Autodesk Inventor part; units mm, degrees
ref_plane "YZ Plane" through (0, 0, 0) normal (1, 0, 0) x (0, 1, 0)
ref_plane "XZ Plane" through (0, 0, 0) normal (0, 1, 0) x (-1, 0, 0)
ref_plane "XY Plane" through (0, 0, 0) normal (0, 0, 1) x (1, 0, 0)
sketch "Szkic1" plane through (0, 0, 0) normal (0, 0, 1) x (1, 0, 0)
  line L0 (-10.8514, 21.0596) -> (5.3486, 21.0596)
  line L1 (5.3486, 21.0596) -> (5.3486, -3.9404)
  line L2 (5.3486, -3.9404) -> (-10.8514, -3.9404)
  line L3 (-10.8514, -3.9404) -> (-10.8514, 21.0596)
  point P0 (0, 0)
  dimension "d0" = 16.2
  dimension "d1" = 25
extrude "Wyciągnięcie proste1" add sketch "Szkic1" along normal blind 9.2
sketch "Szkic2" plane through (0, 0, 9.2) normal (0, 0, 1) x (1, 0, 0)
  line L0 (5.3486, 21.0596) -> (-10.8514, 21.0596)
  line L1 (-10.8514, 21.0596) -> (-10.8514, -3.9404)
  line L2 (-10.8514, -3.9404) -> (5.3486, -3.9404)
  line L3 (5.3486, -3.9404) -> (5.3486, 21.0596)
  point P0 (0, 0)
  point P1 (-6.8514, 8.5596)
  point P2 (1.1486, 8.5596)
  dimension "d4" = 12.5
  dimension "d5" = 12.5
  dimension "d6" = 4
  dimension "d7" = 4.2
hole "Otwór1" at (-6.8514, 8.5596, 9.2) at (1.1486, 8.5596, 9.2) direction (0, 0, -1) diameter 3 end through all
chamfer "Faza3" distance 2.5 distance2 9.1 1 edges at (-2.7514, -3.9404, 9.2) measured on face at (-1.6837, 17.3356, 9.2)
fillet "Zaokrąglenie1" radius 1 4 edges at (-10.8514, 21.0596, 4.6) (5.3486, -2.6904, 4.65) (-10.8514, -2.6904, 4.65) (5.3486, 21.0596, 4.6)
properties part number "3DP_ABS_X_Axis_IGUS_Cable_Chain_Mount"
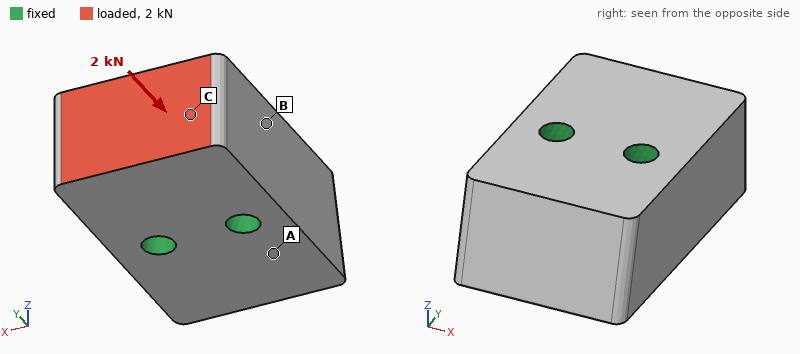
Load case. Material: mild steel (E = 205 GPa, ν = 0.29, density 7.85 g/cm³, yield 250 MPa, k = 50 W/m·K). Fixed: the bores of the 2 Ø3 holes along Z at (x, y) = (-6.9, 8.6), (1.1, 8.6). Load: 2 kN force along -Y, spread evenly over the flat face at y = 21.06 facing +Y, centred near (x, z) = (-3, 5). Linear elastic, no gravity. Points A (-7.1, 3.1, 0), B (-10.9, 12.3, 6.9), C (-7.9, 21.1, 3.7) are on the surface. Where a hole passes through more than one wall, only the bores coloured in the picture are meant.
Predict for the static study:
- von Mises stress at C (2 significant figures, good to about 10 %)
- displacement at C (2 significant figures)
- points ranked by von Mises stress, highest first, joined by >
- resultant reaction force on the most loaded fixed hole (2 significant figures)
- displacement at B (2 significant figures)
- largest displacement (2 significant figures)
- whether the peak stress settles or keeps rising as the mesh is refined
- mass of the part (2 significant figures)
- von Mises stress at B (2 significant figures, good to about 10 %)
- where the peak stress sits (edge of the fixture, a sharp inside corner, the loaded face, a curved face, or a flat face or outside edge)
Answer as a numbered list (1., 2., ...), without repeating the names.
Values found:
1. 12 MPa
2. 0.81 µm
3. C > B > A
4. 1.0 kN
5. 0.32 µm
6. 0.89 µm
7. keeps rising
8. 27 g
9. 8.3 MPa
10. edge of the fixture
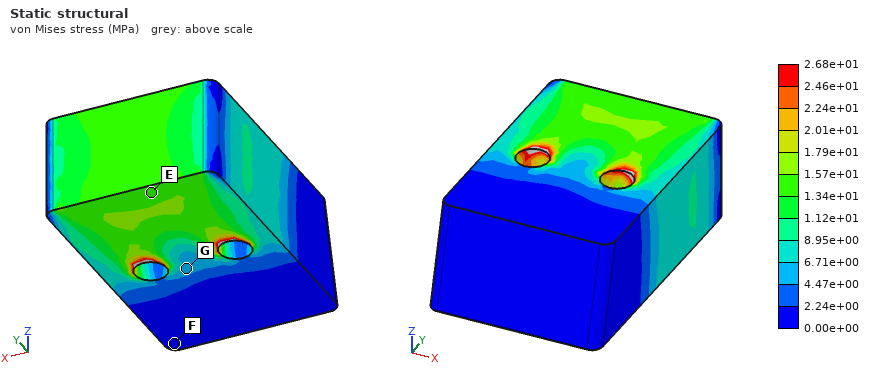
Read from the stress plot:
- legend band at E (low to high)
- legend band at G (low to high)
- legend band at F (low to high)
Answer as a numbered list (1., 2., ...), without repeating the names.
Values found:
1. 1.34e+01 to 1.57e+01 MPa
2. 4.47e+00 to 6.71e+00 MPa
3. 0.00e+00 to 2.24e+00 MPa
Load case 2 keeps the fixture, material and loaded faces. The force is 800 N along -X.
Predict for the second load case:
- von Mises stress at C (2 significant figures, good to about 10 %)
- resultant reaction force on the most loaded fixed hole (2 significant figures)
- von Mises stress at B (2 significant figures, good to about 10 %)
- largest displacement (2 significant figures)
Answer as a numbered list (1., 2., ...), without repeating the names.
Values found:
1. 12 MPa
2. 1.0 kN
3. 15 MPa
4. 2.1 µm
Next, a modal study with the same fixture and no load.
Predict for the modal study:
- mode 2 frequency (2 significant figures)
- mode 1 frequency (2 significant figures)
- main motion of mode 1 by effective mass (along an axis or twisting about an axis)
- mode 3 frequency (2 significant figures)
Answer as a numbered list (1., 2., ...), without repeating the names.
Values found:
1. 45 kHz
2. 38 kHz
3. along Z
4. 46 kHz
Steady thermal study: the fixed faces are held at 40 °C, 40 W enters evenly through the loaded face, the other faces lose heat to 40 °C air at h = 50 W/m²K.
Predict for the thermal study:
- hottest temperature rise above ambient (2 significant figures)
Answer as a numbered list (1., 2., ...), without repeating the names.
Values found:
1. 66 K
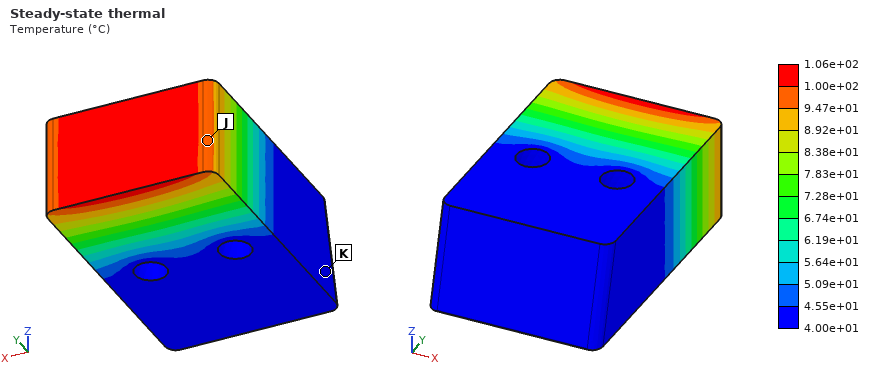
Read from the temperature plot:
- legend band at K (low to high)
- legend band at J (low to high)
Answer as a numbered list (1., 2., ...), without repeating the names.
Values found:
1. 4.00e+01 to 4.55e+01 °C
2. 9.47e+01 to 1.00e+02 °C
